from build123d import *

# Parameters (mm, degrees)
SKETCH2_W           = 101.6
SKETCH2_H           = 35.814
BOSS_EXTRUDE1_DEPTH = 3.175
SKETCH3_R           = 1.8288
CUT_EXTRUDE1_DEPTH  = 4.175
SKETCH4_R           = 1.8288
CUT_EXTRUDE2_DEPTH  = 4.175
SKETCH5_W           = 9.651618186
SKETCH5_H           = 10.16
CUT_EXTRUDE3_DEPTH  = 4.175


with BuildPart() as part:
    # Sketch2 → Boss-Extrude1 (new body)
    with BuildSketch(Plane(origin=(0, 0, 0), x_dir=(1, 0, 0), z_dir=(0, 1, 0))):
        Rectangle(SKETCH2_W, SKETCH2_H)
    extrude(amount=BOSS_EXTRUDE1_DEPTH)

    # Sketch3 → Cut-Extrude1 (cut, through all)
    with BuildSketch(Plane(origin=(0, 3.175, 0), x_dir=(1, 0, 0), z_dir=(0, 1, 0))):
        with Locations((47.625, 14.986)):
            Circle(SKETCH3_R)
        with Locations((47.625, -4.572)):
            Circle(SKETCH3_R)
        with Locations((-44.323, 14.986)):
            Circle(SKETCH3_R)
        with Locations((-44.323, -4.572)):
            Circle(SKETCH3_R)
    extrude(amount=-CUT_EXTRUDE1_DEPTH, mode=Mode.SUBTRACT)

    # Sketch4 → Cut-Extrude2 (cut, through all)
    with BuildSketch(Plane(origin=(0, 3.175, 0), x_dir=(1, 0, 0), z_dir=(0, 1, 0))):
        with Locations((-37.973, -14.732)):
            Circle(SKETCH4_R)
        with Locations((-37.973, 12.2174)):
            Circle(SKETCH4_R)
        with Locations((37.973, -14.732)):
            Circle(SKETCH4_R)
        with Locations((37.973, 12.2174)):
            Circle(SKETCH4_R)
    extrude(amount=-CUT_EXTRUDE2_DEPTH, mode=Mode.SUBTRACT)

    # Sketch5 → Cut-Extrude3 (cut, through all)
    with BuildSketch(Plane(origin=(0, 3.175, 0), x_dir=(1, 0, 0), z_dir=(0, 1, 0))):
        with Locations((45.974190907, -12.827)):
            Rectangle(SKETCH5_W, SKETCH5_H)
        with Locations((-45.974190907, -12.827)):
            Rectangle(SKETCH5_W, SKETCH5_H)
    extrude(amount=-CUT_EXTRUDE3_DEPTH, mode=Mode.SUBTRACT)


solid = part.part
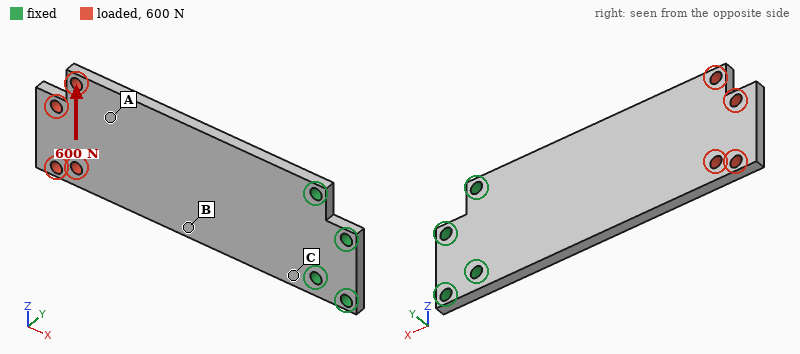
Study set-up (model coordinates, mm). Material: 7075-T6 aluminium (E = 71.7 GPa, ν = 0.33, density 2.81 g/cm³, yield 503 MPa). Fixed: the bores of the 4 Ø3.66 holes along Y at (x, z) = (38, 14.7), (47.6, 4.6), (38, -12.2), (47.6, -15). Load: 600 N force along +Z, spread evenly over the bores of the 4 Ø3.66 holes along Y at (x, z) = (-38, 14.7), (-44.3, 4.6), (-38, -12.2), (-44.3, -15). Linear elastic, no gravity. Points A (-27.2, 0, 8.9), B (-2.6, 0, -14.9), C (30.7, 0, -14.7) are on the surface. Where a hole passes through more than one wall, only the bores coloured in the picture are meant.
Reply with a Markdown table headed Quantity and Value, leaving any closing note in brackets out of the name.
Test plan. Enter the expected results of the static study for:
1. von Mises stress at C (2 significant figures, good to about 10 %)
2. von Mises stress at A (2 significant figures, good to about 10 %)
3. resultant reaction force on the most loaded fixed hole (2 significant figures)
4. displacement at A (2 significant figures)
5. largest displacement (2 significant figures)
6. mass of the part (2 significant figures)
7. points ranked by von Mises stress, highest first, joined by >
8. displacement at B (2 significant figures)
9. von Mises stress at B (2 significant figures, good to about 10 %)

| Quantity | Value |
|---|---|
| von Mises stress at C | 52 MPa |
| von Mises stress at A | 13 MPa |
| resultant reaction force on the most loaded fixed hole | 1.6 kN |
| displacement at A | 0.10 mm |
| largest displacement | 0.16 mm |
| mass of the part | 30 g |
| points ranked by von Mises stress, highest first, joined by > | C > B > A |
| displacement at B | 0.054 mm |
| von Mises stress at B | 29 MPa |
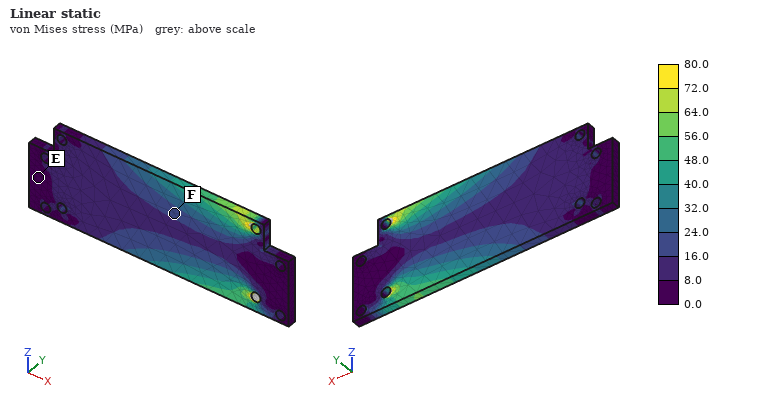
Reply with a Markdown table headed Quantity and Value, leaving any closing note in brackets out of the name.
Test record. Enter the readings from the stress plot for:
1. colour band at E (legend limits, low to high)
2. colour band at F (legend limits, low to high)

| Quantity | Value |
|---|---|
| colour band at E | 0.0 to 8.0 MPa |
| colour band at F | 16.0 to 24.0 MPa |
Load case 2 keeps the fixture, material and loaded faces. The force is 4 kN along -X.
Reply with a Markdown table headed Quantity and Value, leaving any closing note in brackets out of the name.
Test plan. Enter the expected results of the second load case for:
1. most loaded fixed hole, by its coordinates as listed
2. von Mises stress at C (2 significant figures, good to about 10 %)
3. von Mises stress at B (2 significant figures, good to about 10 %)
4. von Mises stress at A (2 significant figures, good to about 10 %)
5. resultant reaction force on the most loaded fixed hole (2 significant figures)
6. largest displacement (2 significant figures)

| Quantity | Value |
|---|---|
| most loaded fixed hole, by its coordinates as listed | (38, -12.2) |
| von Mises stress at C | 51 MPa |
| von Mises stress at B | 45 MPa |
| von Mises stress at A | 27 MPa |
| resultant reaction force on the most loaded fixed hole | 1.9 kN |
| largest displacement | 74 µm |
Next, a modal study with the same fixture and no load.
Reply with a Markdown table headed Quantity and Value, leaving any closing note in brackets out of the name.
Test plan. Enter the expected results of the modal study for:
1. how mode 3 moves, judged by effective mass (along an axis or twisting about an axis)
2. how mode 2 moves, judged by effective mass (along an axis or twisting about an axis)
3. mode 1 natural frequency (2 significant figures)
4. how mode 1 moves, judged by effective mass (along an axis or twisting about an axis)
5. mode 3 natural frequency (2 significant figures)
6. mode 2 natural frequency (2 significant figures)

| Quantity | Value |
|---|---|
| how mode 3 moves, judged by effective mass | along Y |
| how mode 2 moves, judged by effective mass | twisting about X |
| mode 1 natural frequency | 360 Hz |
| how mode 1 moves, judged by effective mass | along Y |
| mode 3 natural frequency | 2200 Hz |
| mode 2 natural frequency | 1800 Hz |
